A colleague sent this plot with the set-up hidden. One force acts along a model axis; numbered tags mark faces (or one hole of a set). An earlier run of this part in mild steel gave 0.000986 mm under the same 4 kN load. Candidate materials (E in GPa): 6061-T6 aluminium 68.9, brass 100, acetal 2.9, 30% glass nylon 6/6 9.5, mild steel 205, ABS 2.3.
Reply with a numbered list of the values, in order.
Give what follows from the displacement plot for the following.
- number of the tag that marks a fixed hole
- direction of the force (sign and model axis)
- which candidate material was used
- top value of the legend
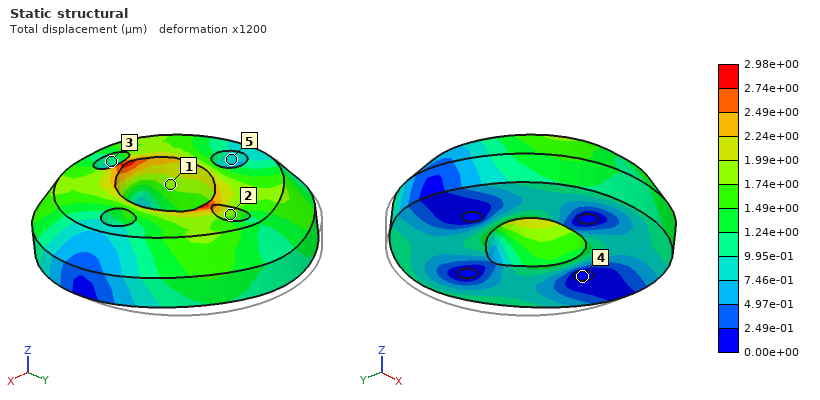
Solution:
1. 4
2. -Y
3. 6061-T6 aluminium
4. 2.98e+00 µm
